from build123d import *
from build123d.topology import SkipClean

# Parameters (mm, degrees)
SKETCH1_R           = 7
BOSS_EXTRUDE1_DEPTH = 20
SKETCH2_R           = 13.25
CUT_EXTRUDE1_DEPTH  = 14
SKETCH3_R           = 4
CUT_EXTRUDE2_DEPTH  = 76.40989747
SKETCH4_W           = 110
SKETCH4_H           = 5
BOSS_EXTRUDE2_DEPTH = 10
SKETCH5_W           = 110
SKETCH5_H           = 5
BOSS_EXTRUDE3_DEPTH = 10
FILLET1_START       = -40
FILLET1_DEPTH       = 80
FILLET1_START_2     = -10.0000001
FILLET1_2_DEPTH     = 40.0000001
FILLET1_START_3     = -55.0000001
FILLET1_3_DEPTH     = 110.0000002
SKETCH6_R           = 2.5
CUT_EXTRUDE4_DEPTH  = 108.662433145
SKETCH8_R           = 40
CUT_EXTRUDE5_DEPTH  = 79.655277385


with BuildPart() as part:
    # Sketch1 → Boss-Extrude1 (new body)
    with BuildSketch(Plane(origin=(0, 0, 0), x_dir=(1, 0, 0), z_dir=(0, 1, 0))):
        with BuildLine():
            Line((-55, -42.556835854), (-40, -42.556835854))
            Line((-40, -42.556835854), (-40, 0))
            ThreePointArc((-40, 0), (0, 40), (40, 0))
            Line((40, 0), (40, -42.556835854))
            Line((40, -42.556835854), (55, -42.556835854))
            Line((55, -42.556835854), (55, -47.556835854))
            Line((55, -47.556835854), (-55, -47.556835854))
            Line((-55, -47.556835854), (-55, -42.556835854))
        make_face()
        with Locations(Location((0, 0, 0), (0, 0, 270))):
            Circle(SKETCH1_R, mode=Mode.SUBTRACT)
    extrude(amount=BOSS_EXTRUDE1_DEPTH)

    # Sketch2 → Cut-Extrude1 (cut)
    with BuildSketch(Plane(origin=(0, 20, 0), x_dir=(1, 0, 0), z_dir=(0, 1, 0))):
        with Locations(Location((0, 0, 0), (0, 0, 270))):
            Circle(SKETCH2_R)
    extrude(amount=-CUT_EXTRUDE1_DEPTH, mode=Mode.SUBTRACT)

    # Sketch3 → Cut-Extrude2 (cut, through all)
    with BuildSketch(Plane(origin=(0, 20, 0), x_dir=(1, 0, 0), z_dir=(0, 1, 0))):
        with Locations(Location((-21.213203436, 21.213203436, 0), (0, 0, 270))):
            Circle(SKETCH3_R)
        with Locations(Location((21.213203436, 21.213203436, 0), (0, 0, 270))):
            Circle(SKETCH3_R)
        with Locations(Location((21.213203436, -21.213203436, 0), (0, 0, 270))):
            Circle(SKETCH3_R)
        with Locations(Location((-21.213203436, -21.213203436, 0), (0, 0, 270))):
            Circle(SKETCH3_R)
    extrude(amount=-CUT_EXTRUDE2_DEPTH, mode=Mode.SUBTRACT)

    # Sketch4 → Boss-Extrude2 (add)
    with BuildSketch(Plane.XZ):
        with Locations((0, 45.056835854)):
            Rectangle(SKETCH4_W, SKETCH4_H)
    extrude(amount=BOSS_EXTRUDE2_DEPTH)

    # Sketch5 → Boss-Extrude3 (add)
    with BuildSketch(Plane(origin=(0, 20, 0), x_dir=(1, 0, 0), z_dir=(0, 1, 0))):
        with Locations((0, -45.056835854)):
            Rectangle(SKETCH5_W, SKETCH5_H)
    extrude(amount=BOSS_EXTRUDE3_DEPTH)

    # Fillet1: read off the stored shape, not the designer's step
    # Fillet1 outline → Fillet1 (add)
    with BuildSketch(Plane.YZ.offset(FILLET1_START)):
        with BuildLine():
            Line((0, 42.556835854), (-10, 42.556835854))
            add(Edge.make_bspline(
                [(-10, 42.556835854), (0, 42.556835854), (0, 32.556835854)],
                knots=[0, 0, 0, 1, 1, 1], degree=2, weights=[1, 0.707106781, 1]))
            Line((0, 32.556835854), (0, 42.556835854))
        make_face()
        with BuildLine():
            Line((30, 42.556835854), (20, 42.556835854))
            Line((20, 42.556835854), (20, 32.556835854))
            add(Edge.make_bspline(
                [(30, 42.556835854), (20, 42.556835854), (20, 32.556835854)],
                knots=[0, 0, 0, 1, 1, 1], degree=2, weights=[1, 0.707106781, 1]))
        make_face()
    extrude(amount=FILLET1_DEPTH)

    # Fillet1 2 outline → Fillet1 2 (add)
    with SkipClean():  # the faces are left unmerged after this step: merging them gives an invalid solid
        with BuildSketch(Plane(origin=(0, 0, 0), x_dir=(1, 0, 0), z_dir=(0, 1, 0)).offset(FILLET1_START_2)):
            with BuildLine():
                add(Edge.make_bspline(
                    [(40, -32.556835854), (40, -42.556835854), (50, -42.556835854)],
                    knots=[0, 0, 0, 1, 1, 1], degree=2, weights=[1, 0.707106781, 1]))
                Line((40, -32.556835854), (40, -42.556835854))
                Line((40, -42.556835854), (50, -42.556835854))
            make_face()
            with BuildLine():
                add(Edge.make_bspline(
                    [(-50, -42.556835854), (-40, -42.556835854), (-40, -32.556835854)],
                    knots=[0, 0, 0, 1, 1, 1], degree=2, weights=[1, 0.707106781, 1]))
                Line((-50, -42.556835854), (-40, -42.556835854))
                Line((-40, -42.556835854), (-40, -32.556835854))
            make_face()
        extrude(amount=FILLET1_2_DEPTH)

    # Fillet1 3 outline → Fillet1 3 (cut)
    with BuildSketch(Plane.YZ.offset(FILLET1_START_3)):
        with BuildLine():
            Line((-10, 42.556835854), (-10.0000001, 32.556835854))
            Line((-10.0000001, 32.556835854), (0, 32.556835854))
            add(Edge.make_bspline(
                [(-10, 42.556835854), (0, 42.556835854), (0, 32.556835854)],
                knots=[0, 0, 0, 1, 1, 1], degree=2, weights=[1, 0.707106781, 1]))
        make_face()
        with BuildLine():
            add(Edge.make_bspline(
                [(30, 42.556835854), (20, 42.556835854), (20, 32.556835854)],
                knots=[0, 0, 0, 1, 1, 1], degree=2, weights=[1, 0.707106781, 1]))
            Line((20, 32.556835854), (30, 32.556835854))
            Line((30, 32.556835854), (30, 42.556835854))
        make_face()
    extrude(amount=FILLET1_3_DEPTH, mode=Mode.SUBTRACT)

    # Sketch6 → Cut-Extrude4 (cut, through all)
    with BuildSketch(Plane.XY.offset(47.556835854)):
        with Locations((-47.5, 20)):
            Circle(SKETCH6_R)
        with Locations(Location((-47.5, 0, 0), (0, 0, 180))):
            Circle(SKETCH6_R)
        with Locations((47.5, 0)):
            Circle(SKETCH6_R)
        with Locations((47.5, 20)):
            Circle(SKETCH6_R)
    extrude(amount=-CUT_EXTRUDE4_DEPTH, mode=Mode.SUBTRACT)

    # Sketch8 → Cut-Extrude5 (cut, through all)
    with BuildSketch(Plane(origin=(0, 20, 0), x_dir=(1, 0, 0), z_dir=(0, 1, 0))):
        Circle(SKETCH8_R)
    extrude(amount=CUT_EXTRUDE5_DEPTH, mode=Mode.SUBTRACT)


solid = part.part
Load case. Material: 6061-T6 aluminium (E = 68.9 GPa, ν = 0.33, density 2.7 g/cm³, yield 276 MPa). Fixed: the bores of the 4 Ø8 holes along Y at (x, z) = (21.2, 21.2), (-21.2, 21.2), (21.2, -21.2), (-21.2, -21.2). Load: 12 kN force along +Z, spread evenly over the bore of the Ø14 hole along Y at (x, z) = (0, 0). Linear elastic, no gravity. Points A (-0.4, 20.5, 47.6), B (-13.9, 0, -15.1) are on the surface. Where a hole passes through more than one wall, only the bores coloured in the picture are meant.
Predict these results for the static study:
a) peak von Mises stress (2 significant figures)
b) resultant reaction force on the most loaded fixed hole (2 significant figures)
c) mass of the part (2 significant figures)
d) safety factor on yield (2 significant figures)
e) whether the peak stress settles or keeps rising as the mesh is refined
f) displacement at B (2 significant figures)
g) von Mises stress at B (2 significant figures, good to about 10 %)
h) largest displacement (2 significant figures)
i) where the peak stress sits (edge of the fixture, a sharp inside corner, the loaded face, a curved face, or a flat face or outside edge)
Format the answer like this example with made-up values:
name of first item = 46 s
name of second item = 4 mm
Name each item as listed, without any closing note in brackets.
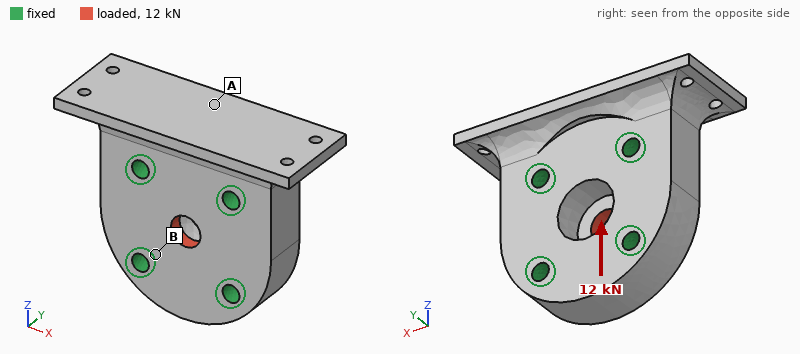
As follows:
peak von Mises stress = 83 MPa
resultant reaction force on the most loaded fixed hole = 3.2 kN
mass of the part = 360 g
safety factor on yield = 3.3
whether the peak stress settles or keeps rising as the mesh is refined = settles
displacement at B = 2.3 µm
von Mises stress at B = 24 MPa
largest displacement = 12 µm
where the peak stress sits = the loaded face
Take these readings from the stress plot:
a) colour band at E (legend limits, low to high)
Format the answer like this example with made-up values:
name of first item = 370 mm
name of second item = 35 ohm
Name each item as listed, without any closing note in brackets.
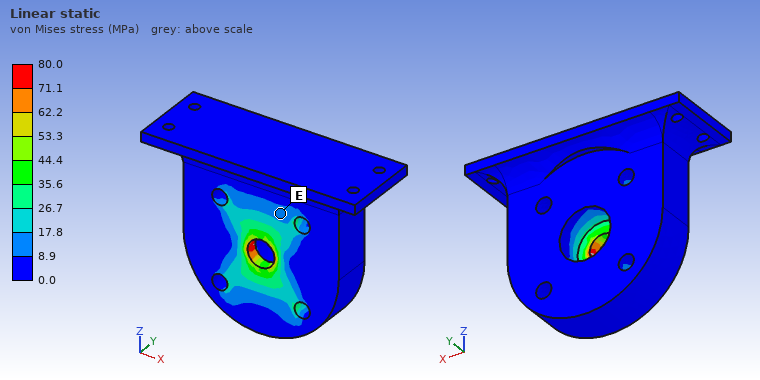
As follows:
colour band at E = 8.9 to 17.8 MPa
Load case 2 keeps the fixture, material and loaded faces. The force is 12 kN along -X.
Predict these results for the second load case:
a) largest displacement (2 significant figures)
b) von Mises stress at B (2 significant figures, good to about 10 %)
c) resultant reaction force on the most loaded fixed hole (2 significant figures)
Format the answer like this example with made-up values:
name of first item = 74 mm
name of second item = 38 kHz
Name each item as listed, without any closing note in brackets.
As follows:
largest displacement = 12 µm
von Mises stress at B = 23 MPa
resultant reaction force on the most loaded fixed hole = 3.3 kN
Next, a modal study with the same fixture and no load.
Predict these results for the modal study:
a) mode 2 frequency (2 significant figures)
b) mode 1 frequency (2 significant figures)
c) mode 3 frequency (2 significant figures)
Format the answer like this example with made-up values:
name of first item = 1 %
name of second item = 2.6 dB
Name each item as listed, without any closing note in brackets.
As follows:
mode 2 frequency = 10 kHz
mode 1 frequency = 10000 Hz
mode 3 frequency = 13 kHz
